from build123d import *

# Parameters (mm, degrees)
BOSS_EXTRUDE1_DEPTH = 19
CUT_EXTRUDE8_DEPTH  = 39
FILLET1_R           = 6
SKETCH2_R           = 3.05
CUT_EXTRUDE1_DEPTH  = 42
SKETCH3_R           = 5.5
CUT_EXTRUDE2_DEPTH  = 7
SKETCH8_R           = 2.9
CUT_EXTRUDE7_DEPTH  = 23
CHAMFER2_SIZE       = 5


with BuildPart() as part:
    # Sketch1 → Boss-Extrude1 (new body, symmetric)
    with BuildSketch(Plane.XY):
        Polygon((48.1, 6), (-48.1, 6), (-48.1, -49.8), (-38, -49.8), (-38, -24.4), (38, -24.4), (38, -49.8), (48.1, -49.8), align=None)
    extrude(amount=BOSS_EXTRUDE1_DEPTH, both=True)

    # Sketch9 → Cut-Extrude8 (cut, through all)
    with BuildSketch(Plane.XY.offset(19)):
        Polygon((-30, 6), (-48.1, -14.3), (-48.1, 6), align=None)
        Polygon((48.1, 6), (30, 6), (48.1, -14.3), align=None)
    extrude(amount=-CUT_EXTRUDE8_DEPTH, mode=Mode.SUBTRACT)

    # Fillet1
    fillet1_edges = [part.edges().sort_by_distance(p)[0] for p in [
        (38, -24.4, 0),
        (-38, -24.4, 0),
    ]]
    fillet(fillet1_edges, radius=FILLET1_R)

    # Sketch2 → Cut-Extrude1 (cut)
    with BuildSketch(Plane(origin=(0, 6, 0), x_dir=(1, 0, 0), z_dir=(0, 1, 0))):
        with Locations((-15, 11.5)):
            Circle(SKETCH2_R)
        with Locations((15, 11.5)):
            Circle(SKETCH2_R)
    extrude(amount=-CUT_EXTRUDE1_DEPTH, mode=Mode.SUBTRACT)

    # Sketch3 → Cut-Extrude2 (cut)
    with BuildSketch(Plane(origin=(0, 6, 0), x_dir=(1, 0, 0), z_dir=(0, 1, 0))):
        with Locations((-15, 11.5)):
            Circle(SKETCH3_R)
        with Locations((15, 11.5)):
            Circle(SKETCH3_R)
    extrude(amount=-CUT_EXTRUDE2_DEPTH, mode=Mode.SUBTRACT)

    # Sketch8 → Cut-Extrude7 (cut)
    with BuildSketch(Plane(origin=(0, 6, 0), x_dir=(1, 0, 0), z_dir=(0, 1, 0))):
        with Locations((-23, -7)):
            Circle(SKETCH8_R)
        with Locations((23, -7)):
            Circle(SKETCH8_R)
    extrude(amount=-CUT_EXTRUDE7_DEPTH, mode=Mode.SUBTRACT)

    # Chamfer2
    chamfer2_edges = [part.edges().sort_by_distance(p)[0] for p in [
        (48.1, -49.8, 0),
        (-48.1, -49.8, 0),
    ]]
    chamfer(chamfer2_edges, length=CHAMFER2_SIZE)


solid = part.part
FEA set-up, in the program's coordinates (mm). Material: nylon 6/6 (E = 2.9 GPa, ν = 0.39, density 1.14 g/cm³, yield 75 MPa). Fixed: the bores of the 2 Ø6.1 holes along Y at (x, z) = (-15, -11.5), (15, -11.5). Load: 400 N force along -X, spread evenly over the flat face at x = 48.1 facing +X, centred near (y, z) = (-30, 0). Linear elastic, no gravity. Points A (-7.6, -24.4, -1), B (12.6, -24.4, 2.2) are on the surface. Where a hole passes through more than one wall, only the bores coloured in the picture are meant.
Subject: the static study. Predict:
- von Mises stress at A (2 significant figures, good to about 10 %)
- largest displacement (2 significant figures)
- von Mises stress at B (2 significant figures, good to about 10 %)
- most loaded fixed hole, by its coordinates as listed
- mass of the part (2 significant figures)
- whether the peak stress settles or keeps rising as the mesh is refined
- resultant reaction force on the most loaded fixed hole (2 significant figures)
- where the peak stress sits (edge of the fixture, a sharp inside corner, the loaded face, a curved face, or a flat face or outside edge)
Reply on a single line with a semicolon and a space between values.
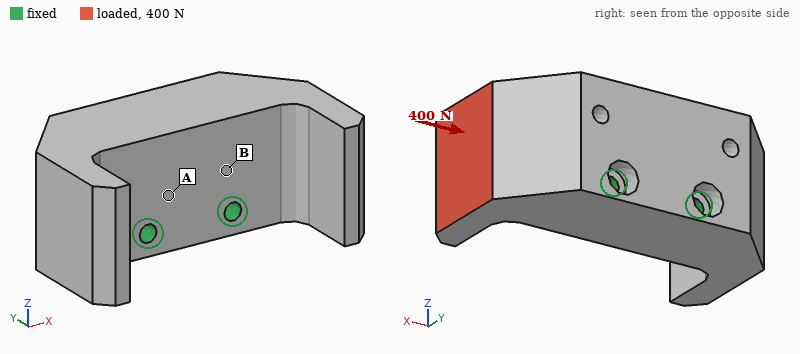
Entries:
0.63 MPa; 0.14 mm; 1.4 MPa; (15, -11.5); 130 g; keeps rising; 340 N; edge of the fixture
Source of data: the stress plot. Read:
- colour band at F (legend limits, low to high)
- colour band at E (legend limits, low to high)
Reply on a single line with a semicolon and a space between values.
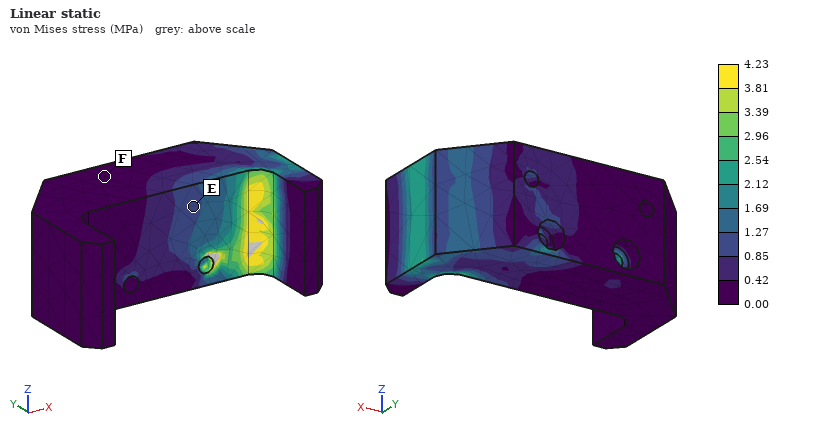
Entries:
0.00 to 0.42 MPa; 0.85 to 1.27 MPa
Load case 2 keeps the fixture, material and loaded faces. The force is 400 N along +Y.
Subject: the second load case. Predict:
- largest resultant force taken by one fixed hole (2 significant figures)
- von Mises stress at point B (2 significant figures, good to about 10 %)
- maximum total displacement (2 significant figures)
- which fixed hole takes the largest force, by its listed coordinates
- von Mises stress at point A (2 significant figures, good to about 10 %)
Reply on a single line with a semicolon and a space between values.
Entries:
530 N; 1.5 MPa; 0.14 mm; (15, -11.5); 0.87 MPa
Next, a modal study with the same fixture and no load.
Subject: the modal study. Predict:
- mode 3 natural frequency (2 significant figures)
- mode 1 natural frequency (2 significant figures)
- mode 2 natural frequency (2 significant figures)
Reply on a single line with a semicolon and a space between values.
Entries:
2200 Hz; 2100 Hz; 2200 Hz
